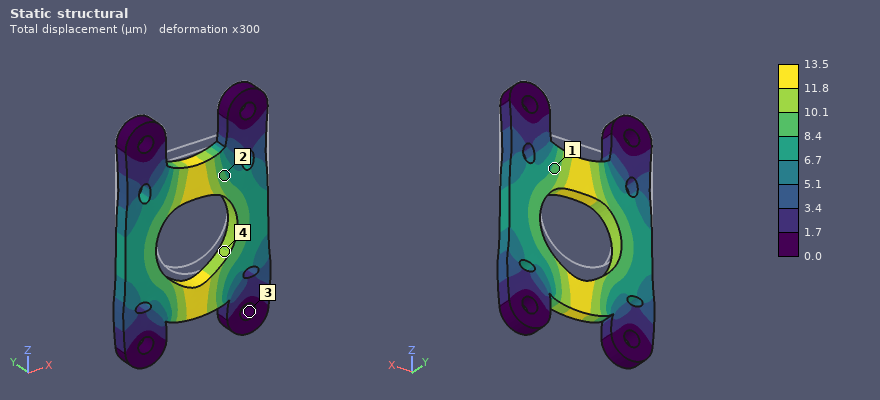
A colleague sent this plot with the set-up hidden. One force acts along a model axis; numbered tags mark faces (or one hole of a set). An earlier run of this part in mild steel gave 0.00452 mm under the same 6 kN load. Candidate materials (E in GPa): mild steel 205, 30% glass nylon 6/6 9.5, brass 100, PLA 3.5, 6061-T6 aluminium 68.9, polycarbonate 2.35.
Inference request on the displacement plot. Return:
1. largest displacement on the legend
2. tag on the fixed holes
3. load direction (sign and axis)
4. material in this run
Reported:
13.5 µm
3
-Z
6061-T6 aluminium
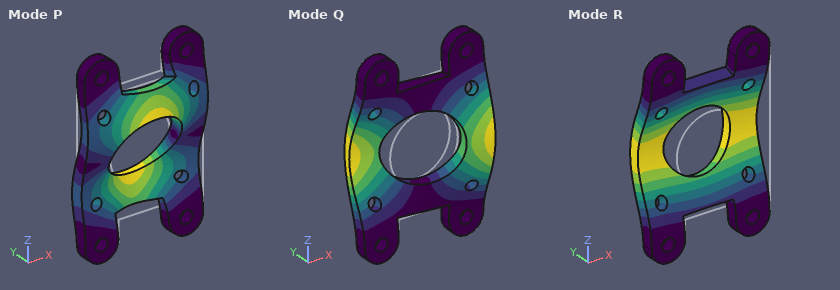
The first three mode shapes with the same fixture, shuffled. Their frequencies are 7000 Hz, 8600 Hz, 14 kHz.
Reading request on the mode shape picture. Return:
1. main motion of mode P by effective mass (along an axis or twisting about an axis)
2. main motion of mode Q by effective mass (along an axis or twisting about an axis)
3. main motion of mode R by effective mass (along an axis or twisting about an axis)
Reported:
twisting about X
twisting about Z
along Y
